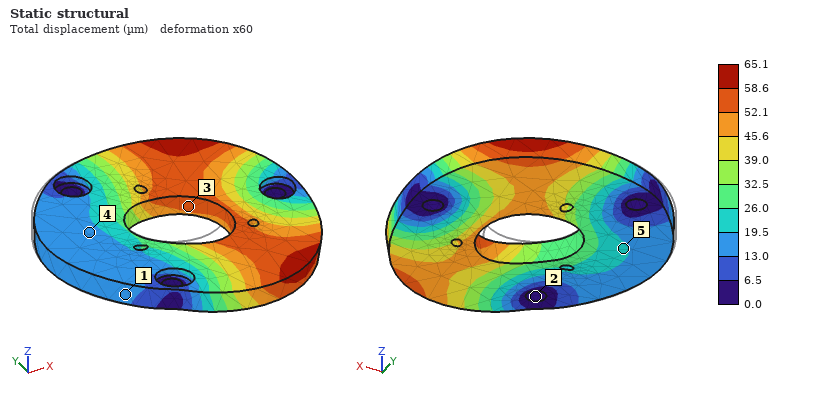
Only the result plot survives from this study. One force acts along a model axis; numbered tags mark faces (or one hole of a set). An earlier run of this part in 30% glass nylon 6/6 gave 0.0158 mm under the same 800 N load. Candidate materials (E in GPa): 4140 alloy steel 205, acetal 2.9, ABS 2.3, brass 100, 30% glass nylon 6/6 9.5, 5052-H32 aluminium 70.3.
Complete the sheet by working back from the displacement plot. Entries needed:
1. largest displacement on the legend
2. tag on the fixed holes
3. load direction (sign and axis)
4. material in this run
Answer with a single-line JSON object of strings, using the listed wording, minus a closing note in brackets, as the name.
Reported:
{"largest displacement on the legend": "65.1 µm", "tag on the fixed holes": "2", "load direction": "-Y", "material in this run": "ABS"}
